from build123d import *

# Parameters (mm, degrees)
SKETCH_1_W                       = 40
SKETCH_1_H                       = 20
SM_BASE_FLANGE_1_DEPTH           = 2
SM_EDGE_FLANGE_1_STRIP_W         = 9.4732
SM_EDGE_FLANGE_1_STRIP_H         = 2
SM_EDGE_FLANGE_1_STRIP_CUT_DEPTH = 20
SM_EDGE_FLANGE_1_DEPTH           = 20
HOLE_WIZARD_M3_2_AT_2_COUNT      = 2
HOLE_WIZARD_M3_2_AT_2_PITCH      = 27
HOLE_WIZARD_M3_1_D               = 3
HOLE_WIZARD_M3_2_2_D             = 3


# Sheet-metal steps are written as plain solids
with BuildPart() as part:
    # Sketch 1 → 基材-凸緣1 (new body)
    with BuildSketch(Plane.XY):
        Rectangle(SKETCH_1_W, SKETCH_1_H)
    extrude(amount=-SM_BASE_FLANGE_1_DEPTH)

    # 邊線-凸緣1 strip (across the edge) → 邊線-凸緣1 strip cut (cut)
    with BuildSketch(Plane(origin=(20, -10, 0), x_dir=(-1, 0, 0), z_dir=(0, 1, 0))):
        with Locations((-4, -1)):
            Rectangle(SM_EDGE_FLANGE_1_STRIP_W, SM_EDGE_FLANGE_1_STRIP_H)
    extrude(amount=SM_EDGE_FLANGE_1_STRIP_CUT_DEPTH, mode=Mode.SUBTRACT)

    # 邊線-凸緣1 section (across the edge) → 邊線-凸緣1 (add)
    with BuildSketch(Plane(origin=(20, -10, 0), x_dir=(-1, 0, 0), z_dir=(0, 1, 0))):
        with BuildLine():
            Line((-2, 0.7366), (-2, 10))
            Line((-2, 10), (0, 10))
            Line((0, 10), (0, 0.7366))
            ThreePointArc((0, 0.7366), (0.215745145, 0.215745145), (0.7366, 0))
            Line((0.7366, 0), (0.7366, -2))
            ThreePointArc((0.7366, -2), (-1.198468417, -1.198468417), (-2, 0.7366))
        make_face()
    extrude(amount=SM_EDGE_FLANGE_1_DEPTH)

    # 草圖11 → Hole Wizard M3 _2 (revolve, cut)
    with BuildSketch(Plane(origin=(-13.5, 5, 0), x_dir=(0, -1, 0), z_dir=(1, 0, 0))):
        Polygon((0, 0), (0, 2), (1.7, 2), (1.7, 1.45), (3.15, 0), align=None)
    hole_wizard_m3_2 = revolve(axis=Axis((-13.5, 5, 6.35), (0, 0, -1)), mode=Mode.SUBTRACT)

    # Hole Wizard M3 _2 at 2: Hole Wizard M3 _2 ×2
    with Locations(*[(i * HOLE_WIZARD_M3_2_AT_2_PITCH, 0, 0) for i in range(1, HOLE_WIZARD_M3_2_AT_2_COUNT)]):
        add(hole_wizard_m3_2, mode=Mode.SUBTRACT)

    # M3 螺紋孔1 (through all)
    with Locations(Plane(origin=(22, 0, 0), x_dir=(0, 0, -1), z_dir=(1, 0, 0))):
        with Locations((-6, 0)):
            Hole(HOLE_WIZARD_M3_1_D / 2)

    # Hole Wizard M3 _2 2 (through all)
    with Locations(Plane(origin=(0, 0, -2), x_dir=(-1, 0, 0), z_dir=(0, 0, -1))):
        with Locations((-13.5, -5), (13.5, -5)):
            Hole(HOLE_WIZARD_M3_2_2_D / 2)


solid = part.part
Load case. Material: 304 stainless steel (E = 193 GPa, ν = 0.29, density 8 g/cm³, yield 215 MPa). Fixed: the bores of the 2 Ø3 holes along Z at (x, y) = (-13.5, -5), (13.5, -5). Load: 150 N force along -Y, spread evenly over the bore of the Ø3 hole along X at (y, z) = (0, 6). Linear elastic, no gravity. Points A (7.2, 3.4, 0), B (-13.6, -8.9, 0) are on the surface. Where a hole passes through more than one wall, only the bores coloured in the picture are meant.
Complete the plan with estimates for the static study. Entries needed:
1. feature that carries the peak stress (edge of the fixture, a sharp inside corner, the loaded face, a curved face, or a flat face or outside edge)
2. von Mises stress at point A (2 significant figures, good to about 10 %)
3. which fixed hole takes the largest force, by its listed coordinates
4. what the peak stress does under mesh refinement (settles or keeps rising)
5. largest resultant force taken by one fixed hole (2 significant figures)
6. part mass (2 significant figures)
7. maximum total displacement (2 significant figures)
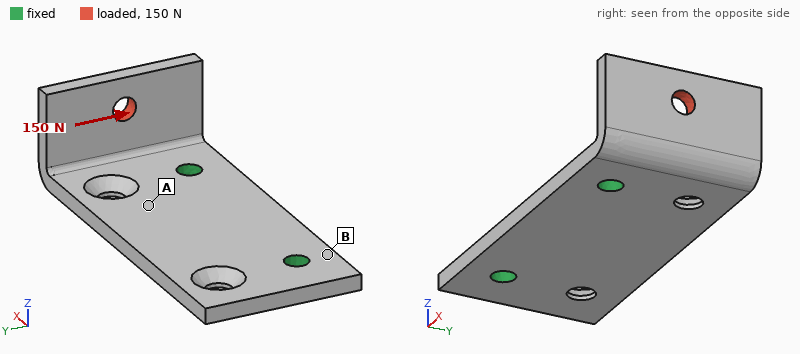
edge of the fixture
21 MPa
(13.5, -5)
keeps rising
180 N
16 g
39 µm
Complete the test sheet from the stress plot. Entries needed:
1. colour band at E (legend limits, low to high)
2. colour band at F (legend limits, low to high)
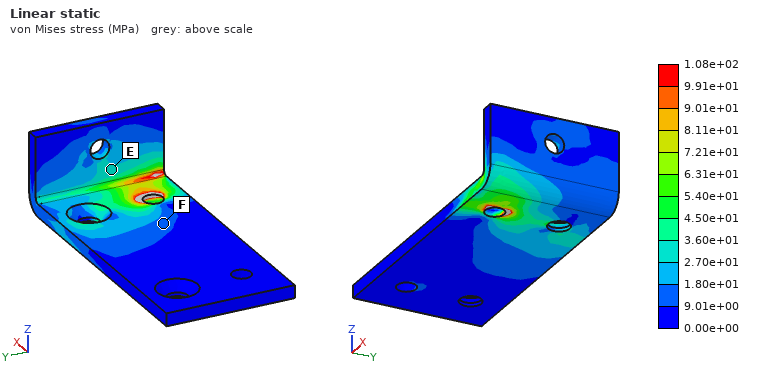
2.70e+01 to 3.60e+01 MPa
9.01e+00 to 1.80e+01 MPa
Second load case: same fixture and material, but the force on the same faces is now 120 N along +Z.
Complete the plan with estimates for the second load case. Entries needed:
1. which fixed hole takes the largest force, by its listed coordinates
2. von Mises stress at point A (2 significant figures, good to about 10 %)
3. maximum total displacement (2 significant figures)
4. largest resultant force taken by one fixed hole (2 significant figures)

(13.5, -5)
15 MPa
35 µm
130 N
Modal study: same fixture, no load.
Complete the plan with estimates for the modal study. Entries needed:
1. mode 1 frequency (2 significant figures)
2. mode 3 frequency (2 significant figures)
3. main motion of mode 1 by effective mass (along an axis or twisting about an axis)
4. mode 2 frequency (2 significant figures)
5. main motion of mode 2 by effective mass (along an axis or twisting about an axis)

4900 Hz
7900 Hz
along Z
6000 Hz
along Z
